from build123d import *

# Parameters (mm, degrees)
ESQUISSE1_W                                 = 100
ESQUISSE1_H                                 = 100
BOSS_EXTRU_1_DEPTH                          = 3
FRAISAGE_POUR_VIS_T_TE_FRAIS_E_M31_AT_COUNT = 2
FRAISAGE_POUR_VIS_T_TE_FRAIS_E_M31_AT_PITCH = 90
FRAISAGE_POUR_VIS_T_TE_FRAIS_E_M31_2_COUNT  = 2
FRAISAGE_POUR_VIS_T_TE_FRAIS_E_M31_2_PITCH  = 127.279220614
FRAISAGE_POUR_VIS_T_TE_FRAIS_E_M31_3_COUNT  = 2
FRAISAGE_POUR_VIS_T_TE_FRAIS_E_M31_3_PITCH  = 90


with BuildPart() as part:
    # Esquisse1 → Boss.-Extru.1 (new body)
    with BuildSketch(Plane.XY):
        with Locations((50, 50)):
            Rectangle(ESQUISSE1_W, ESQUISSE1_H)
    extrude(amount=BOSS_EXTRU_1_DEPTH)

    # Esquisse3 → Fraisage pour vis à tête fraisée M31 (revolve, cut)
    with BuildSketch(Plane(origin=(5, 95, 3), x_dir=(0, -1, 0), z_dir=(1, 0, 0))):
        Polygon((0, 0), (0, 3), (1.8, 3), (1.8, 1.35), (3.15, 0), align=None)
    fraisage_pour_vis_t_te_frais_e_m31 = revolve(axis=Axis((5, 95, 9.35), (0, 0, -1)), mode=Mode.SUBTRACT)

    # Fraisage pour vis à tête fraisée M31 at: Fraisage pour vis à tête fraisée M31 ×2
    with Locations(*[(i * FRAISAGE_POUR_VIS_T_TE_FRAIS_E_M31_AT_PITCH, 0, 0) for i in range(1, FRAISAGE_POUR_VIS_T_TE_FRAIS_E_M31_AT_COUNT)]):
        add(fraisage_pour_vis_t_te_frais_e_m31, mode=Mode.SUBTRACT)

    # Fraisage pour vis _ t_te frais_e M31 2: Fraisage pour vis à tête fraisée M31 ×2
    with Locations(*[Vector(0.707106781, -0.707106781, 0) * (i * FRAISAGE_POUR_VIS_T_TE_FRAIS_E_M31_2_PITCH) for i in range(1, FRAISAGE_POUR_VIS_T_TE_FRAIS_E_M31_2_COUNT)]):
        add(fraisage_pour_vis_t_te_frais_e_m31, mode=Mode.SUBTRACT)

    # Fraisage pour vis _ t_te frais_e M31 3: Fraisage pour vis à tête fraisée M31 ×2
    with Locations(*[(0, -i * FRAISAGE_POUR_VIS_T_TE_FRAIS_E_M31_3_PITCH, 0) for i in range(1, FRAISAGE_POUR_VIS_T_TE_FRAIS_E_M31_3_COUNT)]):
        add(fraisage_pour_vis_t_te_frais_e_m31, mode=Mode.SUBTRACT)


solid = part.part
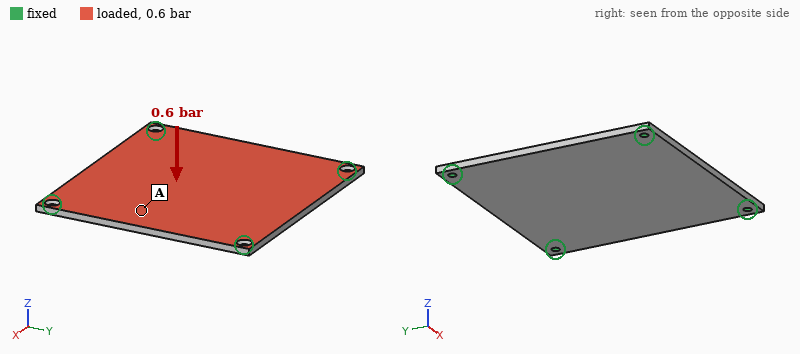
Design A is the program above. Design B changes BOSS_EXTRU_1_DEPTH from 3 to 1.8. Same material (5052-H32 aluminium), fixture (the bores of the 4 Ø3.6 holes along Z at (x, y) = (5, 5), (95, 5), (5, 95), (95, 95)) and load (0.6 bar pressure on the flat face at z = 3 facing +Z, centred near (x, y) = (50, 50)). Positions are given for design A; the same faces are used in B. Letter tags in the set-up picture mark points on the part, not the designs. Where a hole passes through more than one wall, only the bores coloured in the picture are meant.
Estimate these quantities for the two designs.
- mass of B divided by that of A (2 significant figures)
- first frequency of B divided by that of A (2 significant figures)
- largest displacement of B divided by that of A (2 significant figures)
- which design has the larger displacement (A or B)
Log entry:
0.60
0.67
3.8
B
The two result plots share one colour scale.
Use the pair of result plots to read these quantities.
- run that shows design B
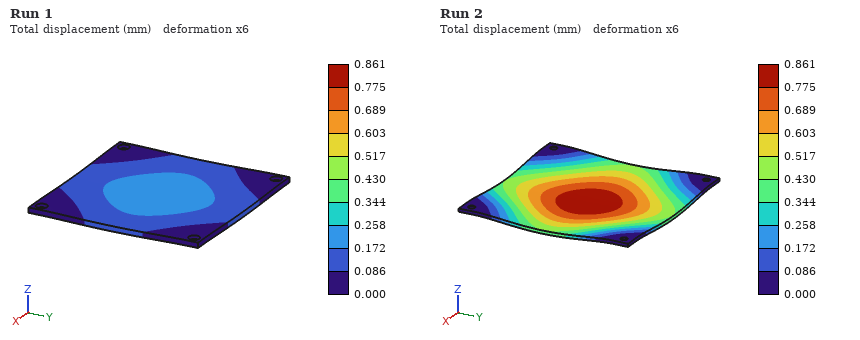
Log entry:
Run 2
